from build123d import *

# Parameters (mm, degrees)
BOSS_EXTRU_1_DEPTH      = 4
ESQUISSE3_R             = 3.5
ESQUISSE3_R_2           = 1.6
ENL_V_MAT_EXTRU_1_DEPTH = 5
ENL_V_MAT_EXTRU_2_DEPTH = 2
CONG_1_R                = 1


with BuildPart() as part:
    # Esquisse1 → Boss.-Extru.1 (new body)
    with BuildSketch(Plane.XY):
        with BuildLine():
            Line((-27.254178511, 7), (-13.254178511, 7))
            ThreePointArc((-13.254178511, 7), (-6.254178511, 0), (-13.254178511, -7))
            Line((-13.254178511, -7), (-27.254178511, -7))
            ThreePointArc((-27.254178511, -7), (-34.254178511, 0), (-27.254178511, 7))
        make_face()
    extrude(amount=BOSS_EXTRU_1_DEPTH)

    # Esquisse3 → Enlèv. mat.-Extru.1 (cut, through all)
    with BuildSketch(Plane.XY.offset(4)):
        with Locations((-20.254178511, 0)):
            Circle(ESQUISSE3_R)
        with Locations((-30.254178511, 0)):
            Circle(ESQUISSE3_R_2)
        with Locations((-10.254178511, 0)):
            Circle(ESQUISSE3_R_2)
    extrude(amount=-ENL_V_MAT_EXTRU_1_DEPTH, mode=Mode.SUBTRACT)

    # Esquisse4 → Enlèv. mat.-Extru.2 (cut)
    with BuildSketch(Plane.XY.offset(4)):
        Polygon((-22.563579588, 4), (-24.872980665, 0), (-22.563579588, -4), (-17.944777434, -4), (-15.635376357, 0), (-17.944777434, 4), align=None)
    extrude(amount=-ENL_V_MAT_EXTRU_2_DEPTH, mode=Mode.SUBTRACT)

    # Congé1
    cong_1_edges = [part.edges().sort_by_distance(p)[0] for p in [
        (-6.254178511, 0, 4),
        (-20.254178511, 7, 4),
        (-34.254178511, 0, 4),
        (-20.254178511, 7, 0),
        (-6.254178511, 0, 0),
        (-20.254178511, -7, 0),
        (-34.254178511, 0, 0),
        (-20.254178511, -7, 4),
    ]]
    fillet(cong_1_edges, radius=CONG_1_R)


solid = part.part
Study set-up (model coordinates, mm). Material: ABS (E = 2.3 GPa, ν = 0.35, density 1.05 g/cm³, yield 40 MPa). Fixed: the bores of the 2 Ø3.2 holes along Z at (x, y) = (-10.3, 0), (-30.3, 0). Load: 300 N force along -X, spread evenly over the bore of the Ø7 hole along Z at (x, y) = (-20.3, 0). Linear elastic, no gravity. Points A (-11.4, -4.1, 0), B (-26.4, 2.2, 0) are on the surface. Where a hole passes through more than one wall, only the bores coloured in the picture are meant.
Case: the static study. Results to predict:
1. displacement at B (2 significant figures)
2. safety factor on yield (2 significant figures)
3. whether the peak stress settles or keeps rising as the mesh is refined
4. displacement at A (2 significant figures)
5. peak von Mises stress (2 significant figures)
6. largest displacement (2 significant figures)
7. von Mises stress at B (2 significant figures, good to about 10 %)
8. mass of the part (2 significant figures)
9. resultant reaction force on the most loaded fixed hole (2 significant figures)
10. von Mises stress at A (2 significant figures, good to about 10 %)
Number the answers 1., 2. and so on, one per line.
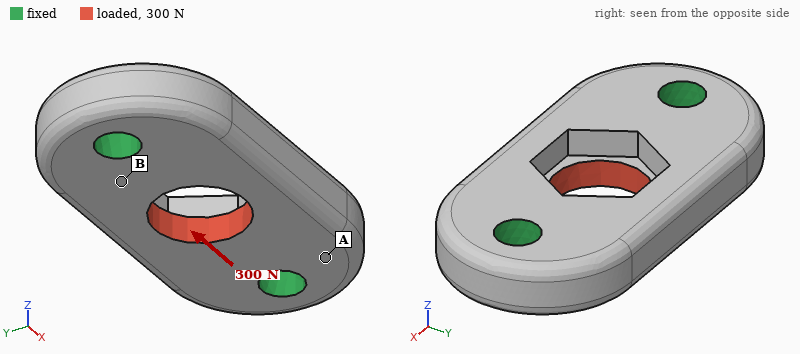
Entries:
1. 11 µm
2. 2.9
3. settles
4. 8.3 µm
5. 14 MPa
6. 24 µm
7. 6.8 MPa
8. 1.2 g
9. 150 N
10. 2.4 MPa
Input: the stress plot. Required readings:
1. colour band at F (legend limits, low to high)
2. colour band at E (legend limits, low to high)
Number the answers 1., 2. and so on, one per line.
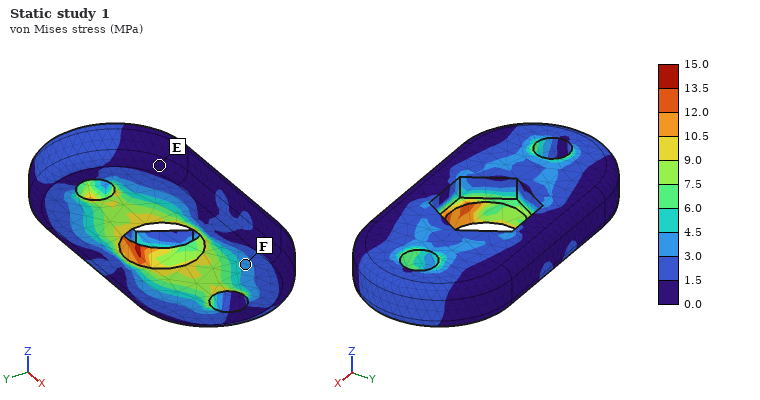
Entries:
1. 3.0 to 4.5 MPa
2. 0.0 to 1.5 MPa
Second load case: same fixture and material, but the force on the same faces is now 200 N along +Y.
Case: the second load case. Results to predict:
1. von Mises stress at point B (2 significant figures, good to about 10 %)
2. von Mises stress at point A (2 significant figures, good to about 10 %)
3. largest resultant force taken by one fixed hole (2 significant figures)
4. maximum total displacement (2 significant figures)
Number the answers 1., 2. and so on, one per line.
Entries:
1. 6.0 MPa
2. 3.1 MPa
3. 100 N
4. 44 µm
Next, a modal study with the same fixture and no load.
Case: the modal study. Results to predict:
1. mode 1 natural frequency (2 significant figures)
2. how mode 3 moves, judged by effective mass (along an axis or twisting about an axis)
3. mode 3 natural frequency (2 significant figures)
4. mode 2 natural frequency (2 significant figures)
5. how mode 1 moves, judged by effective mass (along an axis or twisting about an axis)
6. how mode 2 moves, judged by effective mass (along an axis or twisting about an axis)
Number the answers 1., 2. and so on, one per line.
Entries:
1. 12 kHz
2. along Y
3. 20 kHz
4. 12 kHz
5. twisting about X
6. along Z
